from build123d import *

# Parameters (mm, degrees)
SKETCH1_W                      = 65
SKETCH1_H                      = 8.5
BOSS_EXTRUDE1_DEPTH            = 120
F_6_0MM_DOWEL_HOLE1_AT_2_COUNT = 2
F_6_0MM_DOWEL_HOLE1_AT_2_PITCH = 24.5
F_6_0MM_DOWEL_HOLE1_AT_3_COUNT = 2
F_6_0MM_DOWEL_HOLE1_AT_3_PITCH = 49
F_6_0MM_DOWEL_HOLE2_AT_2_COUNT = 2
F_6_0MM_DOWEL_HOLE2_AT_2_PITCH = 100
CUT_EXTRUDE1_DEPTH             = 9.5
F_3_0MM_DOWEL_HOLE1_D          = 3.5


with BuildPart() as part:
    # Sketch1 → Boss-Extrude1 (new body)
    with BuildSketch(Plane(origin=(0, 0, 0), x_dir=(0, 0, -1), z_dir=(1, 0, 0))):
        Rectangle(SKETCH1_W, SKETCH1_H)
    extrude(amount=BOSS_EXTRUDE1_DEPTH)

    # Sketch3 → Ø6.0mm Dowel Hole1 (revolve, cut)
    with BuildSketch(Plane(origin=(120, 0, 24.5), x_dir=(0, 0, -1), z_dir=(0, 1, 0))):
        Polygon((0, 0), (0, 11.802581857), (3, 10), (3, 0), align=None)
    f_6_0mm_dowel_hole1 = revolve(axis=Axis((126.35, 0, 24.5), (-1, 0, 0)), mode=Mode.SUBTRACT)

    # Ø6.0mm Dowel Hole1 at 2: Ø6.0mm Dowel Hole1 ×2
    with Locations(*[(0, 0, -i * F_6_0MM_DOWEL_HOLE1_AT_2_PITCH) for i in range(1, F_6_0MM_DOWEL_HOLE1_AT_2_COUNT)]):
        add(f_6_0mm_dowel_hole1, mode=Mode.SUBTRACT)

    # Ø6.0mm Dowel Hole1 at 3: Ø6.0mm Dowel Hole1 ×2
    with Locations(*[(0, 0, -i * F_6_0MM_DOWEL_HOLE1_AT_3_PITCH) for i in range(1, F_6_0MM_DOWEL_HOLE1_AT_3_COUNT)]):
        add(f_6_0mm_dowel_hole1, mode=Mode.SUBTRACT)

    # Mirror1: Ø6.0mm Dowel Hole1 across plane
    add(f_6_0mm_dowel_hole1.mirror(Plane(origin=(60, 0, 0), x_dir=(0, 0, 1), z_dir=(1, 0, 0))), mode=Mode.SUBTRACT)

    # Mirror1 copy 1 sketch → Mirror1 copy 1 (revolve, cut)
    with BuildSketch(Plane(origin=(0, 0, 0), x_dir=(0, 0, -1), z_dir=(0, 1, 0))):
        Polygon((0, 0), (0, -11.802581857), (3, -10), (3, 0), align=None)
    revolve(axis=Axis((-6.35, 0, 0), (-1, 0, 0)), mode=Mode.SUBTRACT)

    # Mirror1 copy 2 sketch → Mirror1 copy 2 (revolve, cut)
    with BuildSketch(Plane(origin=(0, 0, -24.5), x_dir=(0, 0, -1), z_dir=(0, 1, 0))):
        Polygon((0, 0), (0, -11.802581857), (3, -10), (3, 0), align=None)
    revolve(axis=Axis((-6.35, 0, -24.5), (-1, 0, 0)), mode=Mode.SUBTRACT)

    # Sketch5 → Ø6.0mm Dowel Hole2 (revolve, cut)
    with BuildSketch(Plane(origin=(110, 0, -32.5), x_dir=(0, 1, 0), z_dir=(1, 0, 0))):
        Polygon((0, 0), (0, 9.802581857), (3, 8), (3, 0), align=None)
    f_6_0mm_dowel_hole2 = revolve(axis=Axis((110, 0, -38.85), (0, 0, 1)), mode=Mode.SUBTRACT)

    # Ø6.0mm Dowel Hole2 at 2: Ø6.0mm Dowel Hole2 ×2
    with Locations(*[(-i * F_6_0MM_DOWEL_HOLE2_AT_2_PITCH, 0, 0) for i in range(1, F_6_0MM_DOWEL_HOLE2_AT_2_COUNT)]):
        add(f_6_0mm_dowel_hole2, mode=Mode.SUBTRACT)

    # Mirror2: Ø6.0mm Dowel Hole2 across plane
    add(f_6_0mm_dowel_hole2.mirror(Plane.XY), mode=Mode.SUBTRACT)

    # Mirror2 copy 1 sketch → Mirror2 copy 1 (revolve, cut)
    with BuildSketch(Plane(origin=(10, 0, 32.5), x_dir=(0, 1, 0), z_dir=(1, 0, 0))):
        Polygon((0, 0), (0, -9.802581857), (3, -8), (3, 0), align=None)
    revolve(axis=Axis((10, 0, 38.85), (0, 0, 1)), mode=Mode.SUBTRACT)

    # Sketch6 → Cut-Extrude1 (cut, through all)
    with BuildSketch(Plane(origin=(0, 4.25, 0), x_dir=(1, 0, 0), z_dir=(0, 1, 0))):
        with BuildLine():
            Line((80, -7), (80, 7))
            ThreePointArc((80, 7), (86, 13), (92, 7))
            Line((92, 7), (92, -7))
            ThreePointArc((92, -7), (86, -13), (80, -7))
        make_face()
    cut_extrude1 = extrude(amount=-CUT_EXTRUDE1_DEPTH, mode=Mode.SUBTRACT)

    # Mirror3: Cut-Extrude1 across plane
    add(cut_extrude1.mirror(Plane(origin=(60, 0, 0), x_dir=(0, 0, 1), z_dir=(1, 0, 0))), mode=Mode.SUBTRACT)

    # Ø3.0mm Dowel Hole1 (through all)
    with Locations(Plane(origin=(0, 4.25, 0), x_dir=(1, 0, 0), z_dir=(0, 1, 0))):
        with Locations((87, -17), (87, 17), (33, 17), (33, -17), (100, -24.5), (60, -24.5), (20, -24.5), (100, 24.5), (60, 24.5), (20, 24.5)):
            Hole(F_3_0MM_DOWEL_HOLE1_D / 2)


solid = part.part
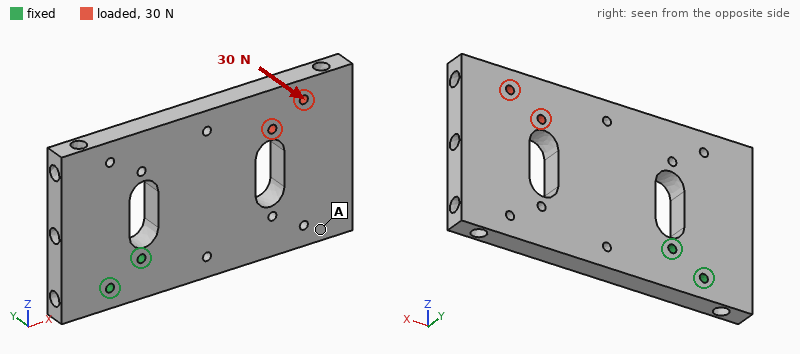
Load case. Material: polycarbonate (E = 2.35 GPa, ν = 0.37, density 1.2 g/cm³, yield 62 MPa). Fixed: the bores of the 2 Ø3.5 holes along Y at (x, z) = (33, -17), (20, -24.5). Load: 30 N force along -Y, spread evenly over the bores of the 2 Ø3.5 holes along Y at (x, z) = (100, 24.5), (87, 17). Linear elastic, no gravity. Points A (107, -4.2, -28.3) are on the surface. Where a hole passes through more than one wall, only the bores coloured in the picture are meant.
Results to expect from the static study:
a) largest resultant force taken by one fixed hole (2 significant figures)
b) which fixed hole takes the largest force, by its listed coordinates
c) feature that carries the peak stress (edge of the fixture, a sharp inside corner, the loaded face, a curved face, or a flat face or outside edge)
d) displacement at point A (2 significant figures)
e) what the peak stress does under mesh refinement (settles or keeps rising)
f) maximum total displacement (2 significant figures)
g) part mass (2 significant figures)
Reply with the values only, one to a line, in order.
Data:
97 N
(33, -17)
edge of the fixture
0.60 mm
keeps rising
1.3 mm
70 g
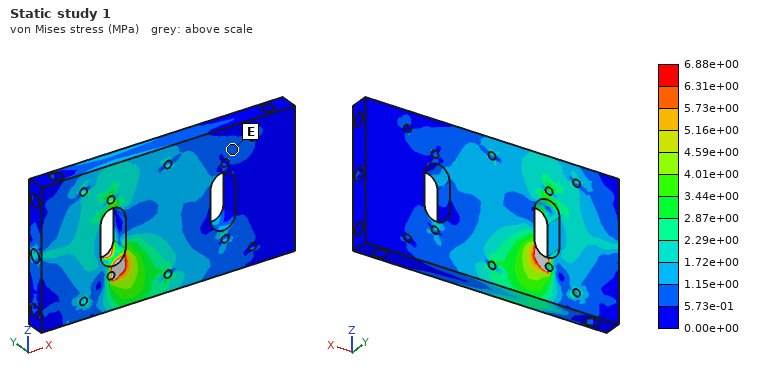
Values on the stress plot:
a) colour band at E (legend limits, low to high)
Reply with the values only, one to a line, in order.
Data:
5.73e-01 to 1.15e+00 MPa
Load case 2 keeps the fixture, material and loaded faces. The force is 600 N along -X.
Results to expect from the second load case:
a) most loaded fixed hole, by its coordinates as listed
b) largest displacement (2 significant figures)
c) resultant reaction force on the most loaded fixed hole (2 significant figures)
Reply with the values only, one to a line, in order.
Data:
(33, -17)
1.4 mm
1.7 kN
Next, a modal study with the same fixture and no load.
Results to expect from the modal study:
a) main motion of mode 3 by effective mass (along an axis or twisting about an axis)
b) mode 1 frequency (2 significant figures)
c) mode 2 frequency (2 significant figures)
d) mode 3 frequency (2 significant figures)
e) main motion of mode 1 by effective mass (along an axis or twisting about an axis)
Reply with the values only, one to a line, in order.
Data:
along Z
190 Hz
410 Hz
500 Hz
along Y
